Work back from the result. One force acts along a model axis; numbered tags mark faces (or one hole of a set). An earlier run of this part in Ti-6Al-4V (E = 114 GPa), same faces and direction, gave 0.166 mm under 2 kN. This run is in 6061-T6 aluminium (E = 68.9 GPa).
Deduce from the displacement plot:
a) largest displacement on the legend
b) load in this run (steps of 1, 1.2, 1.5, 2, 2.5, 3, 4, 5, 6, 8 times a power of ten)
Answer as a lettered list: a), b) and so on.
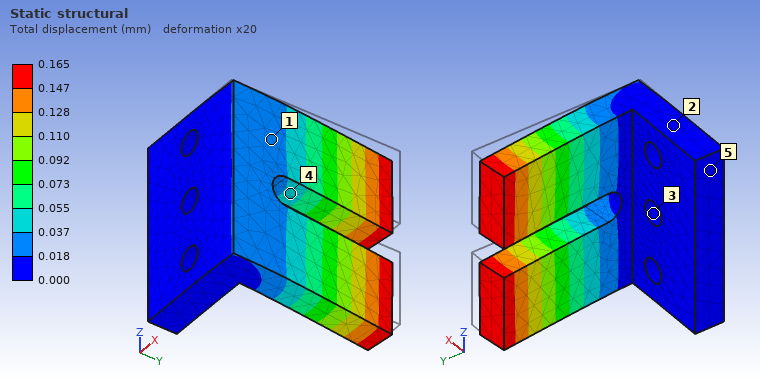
a) 0.165 mm
b) 1.2 kN
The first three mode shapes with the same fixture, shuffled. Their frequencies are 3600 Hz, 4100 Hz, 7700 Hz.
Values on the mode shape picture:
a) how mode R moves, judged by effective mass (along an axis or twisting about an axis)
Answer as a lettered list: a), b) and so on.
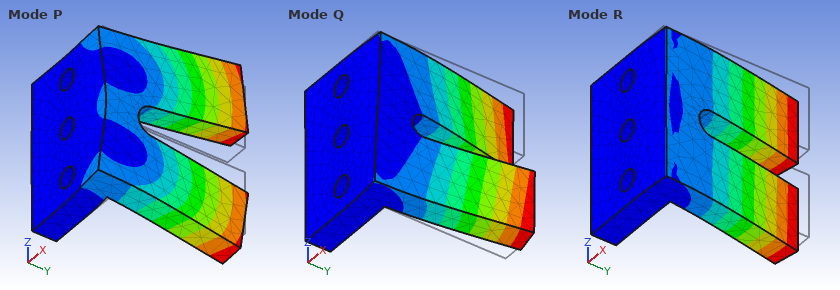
a) along X
